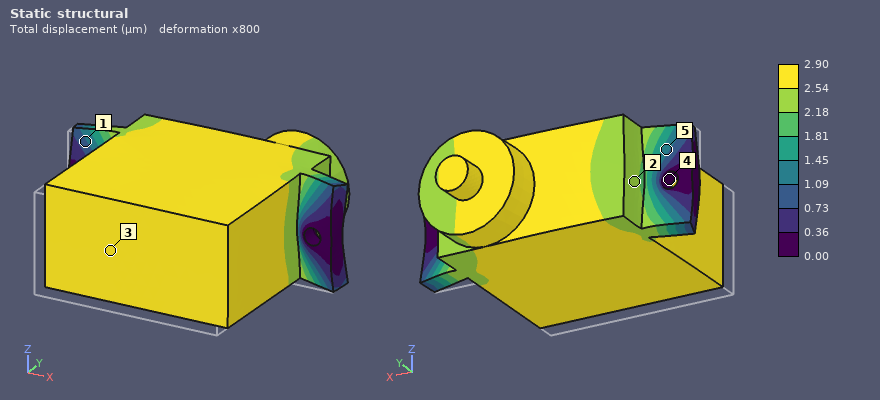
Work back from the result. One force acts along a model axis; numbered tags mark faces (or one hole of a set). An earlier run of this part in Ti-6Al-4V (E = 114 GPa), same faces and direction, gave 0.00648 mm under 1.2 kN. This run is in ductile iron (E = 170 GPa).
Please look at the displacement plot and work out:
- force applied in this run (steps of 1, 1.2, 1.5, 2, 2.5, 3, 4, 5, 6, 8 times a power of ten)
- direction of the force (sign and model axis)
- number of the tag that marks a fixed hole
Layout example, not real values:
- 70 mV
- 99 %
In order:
- 800 N
- +Y
- 4
